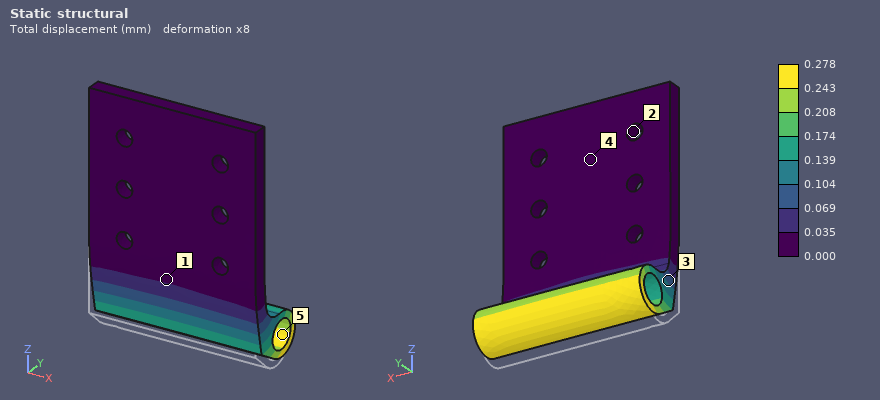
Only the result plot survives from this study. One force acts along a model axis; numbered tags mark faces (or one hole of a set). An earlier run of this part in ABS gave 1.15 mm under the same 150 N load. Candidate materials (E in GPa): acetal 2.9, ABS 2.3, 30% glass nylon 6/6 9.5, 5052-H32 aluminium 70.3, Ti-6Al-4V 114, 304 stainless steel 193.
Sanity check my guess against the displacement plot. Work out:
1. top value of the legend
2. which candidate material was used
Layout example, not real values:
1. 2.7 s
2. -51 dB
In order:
1. 0.278 mm
2. 30% glass nylon 6/6
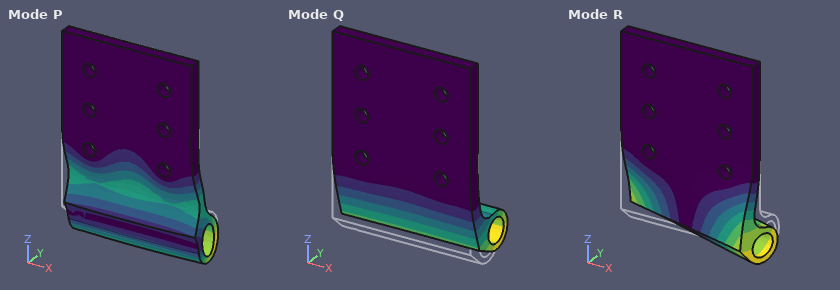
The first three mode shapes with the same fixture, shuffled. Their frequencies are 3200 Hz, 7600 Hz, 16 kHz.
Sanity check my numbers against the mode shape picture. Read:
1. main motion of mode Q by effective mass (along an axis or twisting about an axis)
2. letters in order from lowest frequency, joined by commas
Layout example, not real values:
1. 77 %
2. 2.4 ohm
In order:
1. along Y
2. Q, R, P
